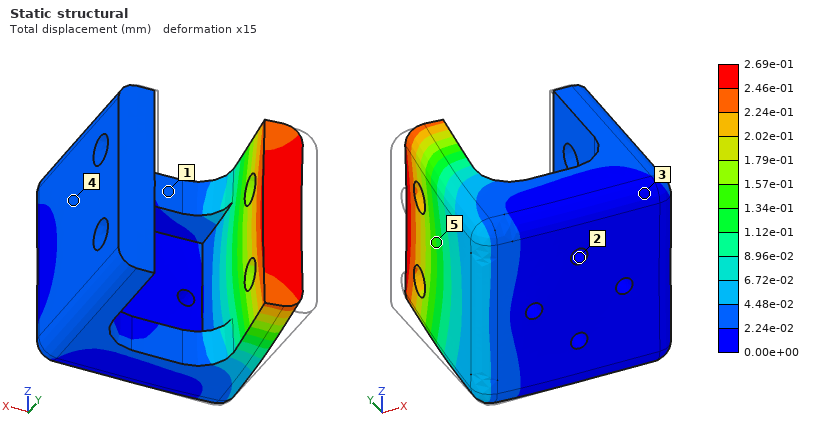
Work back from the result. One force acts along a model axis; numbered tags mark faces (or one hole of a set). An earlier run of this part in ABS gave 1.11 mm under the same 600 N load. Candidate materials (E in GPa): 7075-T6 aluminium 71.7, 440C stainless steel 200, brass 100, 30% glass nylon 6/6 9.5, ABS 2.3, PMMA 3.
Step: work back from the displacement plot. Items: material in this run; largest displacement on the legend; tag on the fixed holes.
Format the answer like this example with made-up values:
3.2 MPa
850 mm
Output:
30% glass nylon 6/6
2.69e-01 mm
2
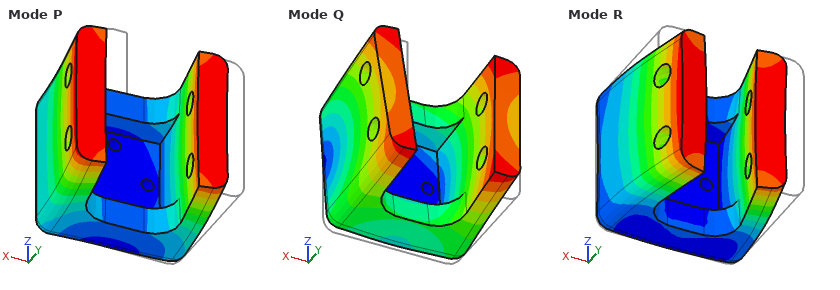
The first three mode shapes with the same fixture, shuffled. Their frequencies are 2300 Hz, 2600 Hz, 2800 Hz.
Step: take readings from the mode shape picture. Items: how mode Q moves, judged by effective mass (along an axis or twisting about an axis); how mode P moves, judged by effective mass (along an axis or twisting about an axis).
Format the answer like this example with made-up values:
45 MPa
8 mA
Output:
along Z
along X
